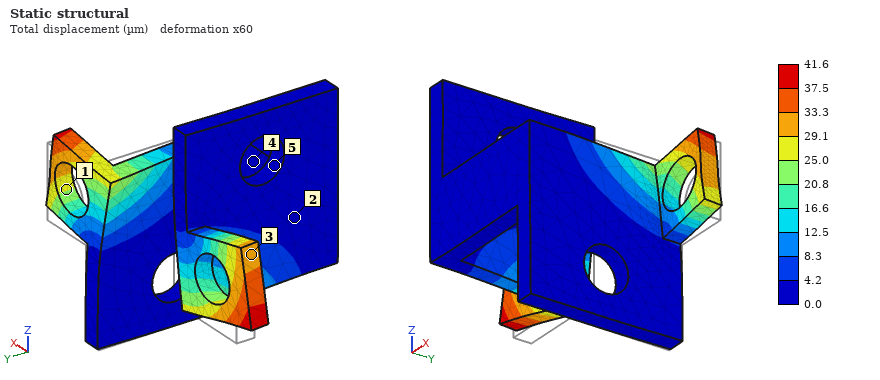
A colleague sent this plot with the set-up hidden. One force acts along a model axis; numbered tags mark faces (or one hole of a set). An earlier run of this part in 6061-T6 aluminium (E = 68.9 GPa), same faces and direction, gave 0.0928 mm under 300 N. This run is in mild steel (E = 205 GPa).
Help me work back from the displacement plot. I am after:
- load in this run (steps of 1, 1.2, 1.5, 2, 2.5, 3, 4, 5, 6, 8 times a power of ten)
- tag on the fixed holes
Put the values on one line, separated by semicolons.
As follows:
400 N; 5
